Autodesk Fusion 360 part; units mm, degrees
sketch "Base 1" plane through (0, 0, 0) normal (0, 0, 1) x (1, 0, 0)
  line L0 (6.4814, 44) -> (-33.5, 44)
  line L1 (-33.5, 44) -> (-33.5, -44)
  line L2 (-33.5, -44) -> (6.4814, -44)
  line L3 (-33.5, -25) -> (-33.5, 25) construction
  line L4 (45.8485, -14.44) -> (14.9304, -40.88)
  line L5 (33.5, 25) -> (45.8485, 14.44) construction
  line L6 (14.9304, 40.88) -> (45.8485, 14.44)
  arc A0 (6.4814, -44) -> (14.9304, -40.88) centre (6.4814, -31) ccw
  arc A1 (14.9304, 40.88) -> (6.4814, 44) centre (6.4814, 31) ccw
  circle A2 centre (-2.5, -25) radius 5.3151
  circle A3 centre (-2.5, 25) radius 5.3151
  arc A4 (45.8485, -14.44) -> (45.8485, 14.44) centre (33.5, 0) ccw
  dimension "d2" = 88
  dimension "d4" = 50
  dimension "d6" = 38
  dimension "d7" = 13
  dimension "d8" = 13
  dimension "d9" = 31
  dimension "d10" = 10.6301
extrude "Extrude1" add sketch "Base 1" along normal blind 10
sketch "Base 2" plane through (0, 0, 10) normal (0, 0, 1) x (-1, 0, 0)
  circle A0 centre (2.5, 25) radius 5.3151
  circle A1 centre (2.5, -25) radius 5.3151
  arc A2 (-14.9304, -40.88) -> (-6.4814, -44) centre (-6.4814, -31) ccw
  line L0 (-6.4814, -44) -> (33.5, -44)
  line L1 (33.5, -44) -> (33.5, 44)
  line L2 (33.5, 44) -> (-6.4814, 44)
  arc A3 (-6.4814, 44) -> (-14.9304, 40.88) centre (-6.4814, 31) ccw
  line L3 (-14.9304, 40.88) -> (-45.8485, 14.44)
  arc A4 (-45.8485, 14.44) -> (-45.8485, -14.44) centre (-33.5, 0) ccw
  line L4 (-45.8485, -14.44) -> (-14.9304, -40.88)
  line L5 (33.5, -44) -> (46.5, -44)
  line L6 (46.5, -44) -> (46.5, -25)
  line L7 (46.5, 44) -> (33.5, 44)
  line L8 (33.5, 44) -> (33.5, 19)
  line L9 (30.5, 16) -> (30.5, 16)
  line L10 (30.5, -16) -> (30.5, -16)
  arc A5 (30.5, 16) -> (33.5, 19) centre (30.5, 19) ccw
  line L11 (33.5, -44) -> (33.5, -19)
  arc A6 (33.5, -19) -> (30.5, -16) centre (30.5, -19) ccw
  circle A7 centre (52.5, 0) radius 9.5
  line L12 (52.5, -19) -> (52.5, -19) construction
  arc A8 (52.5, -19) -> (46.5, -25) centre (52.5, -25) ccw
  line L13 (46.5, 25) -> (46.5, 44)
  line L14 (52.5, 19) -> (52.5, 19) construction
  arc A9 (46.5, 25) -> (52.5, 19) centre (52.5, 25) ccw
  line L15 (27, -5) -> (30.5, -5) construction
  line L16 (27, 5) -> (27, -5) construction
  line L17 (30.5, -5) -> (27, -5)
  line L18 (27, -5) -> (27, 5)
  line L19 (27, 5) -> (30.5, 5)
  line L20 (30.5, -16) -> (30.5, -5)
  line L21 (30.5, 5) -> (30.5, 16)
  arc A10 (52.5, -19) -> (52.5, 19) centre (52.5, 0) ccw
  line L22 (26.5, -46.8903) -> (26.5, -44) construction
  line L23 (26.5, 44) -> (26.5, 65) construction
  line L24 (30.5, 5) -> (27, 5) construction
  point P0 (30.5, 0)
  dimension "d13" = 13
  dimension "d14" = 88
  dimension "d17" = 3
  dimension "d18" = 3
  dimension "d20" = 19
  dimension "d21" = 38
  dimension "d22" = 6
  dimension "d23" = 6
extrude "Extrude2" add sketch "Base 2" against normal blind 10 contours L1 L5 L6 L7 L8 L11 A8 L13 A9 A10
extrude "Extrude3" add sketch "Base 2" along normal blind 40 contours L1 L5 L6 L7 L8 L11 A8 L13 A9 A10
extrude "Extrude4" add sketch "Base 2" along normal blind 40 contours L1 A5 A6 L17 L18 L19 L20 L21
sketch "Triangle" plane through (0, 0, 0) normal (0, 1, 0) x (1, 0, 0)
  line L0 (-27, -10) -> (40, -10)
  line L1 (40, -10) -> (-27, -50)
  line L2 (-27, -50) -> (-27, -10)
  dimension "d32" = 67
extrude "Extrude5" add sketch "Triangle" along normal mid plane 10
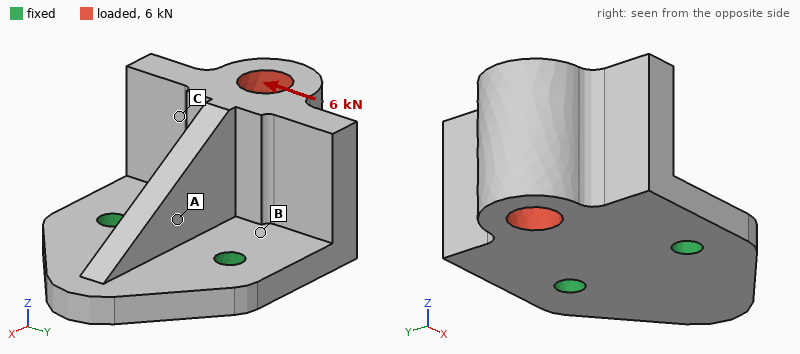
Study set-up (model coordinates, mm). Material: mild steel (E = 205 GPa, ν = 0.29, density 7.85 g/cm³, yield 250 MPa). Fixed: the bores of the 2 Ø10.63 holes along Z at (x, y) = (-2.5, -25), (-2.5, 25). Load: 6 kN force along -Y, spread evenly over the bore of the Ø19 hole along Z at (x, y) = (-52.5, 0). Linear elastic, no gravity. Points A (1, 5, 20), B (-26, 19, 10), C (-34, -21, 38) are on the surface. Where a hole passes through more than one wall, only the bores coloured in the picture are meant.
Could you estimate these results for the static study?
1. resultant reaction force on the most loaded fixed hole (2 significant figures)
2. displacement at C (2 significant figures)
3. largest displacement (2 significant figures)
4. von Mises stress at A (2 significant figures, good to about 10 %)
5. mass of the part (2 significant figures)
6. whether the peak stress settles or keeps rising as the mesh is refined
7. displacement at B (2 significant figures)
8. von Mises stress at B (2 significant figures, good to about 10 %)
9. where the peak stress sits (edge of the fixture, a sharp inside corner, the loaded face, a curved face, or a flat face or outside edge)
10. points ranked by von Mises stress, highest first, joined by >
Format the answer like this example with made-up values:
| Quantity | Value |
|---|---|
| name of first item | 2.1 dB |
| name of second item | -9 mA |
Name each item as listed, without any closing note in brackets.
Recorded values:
| Quantity | Value |
|---|---|
| resultant reaction force on the most loaded fixed hole | 6.5 kN |
| displacement at C | 19 µm |
| largest displacement | 28 µm |
| von Mises stress at A | 15 MPa |
| mass of the part | 1.3 kg |
| whether the peak stress settles or keeps rising as the mesh is refined | keeps rising |
| displacement at B | 6.4 µm |
| von Mises stress at B | 35 MPa |
| where the peak stress sits | edge of the fixture |
| points ranked by von Mises stress, highest first, joined by > | B > A > C |
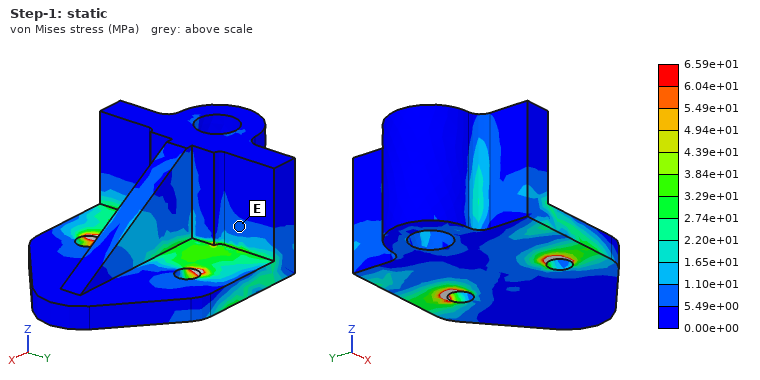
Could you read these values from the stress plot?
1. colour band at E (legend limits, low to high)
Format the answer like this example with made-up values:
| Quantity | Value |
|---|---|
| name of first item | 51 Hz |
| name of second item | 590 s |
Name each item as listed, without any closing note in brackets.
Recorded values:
| Quantity | Value |
|---|---|
| colour band at E | 5.49e+00 to 1.10e+01 MPa |
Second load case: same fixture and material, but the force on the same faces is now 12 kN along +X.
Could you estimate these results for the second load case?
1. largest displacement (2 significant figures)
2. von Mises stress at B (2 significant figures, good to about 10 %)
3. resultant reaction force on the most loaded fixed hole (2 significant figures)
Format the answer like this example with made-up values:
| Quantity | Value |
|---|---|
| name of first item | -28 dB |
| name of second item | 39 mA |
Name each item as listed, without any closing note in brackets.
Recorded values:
| Quantity | Value |
|---|---|
| largest displacement | 0.11 mm |
| von Mises stress at B | 27 MPa |
| resultant reaction force on the most loaded fixed hole | 6.0 kN |
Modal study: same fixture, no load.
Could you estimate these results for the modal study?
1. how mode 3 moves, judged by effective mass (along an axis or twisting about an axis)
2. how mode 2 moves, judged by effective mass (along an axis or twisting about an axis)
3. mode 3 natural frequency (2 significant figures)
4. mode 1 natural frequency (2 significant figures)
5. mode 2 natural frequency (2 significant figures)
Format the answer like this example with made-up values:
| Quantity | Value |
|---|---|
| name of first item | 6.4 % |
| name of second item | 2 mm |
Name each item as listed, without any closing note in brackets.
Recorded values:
| Quantity | Value |
|---|---|
| how mode 3 moves, judged by effective mass | along Z |
| how mode 2 moves, judged by effective mass | along Y |
| mode 3 natural frequency | 5600 Hz |
| mode 1 natural frequency | 1600 Hz |
| mode 2 natural frequency | 2900 Hz |
